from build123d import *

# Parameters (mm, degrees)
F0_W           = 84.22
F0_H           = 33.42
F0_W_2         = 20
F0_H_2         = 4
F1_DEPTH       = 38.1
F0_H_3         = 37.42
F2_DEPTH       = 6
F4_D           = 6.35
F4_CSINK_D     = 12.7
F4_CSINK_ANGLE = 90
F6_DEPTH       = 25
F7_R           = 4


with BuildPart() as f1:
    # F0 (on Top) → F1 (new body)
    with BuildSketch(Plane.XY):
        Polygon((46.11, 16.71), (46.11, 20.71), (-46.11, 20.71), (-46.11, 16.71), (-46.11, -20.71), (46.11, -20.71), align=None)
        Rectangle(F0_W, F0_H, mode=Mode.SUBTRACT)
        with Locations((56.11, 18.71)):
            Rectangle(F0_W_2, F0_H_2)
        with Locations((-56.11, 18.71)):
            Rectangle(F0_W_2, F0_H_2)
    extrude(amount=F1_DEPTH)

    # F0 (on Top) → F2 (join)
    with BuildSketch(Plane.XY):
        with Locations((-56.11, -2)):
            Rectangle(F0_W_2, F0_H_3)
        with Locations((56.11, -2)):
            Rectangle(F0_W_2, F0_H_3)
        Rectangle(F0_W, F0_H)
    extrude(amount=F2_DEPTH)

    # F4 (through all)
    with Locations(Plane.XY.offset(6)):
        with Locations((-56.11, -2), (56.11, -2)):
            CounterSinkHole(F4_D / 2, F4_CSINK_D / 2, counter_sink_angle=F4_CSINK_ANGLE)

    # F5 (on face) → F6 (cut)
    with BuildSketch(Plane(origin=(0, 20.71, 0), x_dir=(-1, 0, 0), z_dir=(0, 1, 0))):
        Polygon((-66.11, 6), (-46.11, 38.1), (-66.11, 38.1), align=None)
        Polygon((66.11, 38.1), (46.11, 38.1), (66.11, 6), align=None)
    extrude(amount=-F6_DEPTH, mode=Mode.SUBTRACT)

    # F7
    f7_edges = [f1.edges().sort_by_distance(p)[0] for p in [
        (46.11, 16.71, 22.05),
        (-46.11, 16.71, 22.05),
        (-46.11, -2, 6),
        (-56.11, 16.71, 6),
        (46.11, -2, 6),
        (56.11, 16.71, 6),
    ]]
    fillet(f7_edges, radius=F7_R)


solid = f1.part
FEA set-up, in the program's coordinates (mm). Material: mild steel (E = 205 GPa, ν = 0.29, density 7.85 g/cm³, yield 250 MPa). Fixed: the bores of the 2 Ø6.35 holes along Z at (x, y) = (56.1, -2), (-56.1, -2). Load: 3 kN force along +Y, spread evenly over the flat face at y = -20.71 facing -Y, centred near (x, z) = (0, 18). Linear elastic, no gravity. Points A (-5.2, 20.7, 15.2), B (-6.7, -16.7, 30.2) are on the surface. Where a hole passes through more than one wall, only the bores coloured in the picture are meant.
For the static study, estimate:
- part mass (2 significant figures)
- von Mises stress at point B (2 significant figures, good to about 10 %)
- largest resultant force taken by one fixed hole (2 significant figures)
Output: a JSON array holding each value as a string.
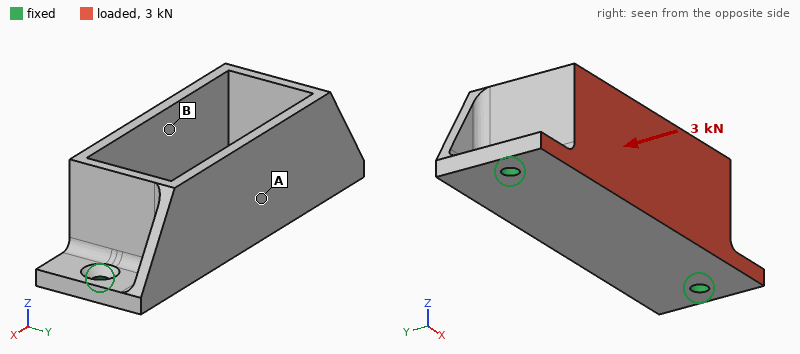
["530 g", "39 MPa", "1.5 kN"]
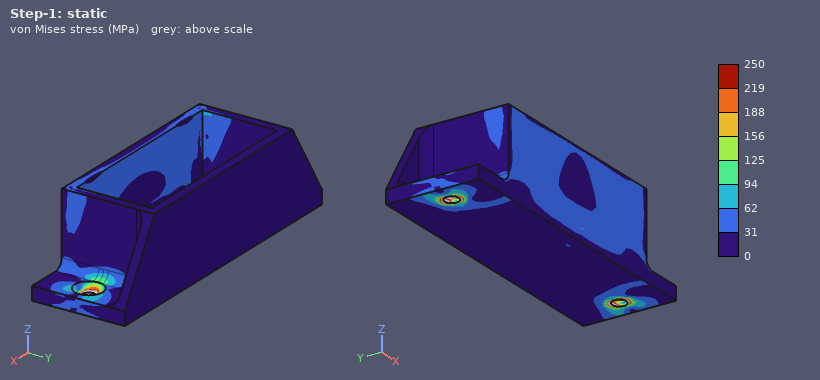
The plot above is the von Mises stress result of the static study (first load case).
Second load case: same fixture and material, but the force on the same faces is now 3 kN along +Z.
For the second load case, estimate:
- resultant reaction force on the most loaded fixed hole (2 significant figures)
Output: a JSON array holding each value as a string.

["2.0 kN"]
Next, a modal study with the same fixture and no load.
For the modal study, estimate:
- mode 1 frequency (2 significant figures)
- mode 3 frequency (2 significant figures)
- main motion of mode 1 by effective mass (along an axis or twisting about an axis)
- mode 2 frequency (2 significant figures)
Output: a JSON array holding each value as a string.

["1400 Hz", "3900 Hz", "along Y", "3000 Hz"]
